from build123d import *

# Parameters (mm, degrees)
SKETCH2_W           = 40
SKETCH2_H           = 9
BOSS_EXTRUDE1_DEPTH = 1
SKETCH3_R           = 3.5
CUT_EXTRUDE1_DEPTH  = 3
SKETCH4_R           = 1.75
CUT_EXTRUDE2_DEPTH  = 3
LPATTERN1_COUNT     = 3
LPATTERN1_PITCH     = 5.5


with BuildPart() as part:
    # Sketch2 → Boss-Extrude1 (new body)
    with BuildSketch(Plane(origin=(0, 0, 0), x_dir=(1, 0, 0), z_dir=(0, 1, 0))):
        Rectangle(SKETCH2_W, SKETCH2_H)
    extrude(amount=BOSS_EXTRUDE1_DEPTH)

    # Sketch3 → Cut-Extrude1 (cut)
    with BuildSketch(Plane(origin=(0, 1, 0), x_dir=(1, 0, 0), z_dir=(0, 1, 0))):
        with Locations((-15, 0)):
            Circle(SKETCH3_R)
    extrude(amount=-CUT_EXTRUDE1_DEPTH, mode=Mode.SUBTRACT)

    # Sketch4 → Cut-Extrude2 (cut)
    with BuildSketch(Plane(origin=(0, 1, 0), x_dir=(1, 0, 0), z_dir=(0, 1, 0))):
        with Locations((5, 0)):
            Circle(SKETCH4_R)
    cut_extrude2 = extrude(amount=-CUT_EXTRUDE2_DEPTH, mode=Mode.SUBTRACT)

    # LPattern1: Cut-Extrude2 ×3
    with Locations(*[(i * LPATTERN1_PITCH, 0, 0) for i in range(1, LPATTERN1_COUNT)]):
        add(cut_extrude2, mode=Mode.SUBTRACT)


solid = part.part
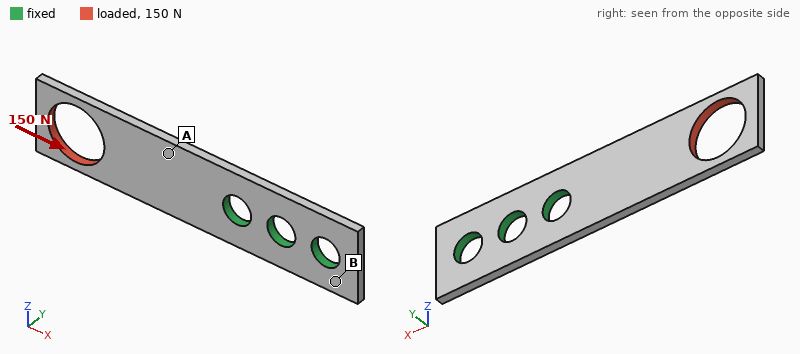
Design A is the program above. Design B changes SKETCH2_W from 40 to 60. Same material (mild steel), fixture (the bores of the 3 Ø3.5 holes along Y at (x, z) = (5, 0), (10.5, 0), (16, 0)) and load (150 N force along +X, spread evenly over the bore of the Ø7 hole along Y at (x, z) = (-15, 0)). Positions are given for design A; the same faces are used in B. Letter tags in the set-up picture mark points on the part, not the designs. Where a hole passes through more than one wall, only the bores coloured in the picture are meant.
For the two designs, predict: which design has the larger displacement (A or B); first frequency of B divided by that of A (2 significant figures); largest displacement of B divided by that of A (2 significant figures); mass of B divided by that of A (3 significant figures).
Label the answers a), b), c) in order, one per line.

a) A
b) 0.38
c) 0.59
d) 1.62
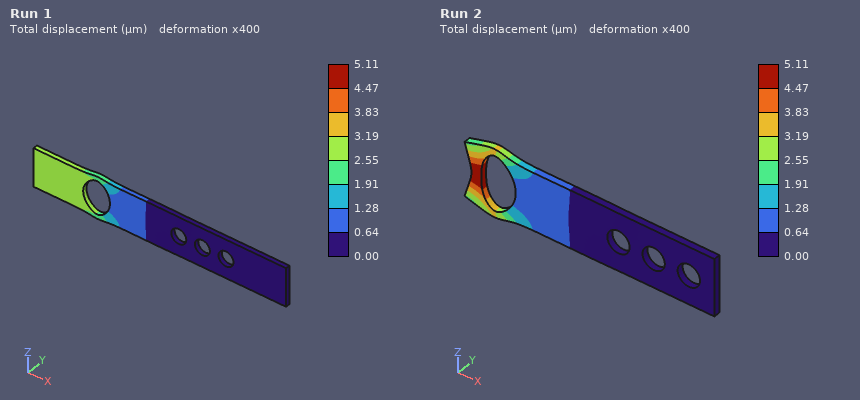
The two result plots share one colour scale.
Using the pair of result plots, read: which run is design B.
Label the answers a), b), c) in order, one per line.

a) Run 1
